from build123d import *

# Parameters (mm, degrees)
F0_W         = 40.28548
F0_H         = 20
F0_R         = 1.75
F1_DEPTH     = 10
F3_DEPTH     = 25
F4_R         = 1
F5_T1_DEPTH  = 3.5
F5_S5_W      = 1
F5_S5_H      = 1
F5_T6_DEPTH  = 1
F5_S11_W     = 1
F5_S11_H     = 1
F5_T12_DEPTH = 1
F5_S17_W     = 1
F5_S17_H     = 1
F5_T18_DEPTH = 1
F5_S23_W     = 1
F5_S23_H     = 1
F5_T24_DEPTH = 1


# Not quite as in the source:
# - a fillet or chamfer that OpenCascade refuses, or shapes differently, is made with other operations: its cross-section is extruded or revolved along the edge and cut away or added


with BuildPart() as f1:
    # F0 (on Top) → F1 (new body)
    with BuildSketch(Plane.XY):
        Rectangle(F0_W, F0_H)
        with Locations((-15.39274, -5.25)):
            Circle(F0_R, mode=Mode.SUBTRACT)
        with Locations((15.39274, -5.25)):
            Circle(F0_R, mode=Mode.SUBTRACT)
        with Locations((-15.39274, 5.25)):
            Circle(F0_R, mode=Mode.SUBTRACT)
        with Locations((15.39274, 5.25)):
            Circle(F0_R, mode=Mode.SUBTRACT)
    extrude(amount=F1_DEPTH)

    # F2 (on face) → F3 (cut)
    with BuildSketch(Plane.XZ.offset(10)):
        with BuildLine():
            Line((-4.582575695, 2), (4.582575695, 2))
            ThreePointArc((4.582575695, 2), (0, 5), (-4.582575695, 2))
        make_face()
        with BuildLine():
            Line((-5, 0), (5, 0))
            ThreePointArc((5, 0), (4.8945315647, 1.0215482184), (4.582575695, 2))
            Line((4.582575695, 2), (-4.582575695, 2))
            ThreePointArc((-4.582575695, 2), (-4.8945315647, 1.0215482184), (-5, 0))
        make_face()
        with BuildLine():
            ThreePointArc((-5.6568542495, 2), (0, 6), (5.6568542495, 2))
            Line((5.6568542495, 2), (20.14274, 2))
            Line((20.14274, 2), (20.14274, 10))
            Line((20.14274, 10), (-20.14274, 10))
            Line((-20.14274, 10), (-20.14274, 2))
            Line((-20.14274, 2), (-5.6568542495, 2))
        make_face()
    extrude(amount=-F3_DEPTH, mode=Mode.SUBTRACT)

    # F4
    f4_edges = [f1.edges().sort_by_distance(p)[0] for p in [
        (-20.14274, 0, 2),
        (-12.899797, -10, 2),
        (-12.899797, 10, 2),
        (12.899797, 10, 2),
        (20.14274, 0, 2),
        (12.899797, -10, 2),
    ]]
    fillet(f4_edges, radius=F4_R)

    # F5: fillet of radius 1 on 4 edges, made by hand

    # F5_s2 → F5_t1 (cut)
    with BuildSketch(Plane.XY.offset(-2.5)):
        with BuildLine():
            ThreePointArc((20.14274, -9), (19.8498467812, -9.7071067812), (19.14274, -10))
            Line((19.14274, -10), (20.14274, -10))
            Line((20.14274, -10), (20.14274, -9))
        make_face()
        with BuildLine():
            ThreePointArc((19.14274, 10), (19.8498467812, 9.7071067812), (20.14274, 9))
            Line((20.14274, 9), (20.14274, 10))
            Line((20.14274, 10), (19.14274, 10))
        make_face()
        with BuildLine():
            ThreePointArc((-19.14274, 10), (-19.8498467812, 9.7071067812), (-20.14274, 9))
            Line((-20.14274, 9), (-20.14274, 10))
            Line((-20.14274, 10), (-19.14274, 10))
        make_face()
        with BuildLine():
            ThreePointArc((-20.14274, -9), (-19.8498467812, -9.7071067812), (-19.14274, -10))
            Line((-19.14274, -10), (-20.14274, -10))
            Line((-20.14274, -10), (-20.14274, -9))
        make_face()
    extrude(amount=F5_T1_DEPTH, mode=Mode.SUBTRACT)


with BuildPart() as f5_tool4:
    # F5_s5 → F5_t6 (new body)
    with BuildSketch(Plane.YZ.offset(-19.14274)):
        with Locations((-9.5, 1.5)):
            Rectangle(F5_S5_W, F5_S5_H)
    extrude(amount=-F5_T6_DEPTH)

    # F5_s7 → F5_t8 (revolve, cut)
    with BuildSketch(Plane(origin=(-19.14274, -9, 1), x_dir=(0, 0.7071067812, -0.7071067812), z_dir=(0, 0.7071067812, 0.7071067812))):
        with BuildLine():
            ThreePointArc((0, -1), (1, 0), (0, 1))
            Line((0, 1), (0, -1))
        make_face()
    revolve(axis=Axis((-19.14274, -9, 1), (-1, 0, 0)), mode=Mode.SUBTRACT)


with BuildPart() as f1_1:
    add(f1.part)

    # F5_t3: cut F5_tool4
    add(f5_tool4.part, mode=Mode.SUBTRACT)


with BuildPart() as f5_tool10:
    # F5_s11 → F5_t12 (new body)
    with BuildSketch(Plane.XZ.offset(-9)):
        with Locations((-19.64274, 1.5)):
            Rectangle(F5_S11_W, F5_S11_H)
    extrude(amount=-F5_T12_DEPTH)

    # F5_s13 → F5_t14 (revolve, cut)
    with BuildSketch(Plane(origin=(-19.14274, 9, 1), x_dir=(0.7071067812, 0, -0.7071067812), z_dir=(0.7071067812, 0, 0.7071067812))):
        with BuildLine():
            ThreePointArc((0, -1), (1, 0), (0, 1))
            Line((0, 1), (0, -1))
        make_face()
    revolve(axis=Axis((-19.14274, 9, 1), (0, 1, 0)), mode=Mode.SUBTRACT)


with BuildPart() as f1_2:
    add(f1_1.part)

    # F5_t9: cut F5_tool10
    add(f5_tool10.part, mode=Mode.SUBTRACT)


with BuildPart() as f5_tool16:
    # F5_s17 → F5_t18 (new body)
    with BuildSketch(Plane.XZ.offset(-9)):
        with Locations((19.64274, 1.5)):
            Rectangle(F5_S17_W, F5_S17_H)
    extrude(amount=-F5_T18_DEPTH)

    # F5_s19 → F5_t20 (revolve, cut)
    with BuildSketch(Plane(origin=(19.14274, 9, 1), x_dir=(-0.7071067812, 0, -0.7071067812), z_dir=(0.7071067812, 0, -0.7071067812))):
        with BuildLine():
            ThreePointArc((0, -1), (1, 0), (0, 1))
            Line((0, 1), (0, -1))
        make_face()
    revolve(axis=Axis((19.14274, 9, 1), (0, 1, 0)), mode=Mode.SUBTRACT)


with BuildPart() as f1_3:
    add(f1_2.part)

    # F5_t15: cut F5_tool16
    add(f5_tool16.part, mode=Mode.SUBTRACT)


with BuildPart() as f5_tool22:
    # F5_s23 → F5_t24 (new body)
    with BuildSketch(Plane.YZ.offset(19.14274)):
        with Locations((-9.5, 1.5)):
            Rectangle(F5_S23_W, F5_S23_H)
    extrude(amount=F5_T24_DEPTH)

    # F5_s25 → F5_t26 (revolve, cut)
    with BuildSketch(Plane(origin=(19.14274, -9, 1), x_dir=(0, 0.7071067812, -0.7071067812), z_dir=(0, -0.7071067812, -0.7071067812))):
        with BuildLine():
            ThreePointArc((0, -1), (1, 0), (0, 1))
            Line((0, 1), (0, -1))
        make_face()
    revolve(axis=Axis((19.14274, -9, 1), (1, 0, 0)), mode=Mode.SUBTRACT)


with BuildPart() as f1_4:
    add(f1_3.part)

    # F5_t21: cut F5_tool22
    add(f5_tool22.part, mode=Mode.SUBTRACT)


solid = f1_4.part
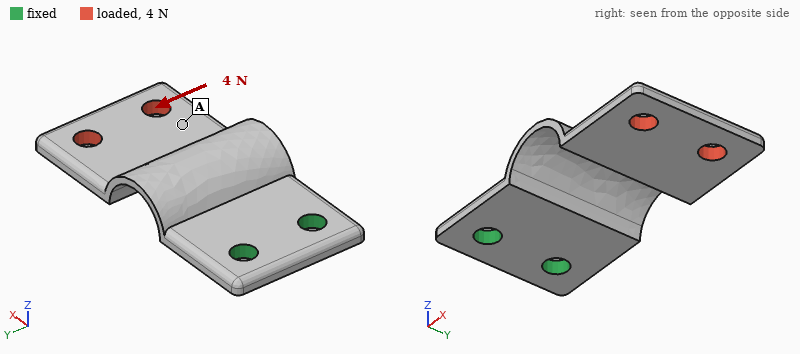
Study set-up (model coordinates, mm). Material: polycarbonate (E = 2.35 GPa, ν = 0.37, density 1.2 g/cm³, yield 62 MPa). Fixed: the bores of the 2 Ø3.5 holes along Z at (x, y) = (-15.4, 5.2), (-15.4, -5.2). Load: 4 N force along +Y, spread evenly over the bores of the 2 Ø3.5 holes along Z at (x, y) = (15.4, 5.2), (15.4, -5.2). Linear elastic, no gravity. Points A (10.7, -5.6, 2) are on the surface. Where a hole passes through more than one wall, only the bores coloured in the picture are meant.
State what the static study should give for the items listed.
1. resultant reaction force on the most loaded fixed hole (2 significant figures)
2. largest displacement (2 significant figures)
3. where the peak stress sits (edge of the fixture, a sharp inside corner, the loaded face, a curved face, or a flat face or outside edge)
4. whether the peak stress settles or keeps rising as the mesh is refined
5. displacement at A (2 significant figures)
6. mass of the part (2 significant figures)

9.8 N
0.44 mm
a sharp inside corner
keeps rising
0.26 mm
1.7 g
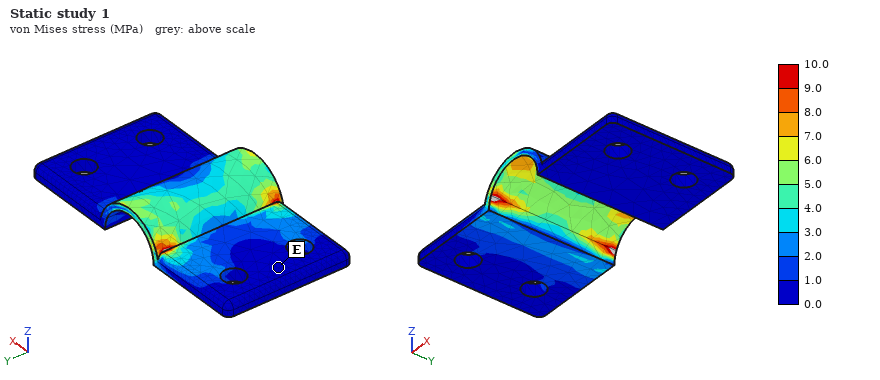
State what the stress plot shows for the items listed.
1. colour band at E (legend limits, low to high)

0.0 to 1.0 MPa
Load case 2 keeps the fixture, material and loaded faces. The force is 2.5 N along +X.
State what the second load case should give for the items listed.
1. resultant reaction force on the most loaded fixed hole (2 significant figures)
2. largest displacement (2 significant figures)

1.3 N
0.51 mm
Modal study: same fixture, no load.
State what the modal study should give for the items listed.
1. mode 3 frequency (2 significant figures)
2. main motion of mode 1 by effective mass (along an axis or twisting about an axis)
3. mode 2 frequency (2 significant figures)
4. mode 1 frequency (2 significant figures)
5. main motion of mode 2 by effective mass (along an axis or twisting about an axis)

1200 Hz
along Z
650 Hz
220 Hz
along Y
